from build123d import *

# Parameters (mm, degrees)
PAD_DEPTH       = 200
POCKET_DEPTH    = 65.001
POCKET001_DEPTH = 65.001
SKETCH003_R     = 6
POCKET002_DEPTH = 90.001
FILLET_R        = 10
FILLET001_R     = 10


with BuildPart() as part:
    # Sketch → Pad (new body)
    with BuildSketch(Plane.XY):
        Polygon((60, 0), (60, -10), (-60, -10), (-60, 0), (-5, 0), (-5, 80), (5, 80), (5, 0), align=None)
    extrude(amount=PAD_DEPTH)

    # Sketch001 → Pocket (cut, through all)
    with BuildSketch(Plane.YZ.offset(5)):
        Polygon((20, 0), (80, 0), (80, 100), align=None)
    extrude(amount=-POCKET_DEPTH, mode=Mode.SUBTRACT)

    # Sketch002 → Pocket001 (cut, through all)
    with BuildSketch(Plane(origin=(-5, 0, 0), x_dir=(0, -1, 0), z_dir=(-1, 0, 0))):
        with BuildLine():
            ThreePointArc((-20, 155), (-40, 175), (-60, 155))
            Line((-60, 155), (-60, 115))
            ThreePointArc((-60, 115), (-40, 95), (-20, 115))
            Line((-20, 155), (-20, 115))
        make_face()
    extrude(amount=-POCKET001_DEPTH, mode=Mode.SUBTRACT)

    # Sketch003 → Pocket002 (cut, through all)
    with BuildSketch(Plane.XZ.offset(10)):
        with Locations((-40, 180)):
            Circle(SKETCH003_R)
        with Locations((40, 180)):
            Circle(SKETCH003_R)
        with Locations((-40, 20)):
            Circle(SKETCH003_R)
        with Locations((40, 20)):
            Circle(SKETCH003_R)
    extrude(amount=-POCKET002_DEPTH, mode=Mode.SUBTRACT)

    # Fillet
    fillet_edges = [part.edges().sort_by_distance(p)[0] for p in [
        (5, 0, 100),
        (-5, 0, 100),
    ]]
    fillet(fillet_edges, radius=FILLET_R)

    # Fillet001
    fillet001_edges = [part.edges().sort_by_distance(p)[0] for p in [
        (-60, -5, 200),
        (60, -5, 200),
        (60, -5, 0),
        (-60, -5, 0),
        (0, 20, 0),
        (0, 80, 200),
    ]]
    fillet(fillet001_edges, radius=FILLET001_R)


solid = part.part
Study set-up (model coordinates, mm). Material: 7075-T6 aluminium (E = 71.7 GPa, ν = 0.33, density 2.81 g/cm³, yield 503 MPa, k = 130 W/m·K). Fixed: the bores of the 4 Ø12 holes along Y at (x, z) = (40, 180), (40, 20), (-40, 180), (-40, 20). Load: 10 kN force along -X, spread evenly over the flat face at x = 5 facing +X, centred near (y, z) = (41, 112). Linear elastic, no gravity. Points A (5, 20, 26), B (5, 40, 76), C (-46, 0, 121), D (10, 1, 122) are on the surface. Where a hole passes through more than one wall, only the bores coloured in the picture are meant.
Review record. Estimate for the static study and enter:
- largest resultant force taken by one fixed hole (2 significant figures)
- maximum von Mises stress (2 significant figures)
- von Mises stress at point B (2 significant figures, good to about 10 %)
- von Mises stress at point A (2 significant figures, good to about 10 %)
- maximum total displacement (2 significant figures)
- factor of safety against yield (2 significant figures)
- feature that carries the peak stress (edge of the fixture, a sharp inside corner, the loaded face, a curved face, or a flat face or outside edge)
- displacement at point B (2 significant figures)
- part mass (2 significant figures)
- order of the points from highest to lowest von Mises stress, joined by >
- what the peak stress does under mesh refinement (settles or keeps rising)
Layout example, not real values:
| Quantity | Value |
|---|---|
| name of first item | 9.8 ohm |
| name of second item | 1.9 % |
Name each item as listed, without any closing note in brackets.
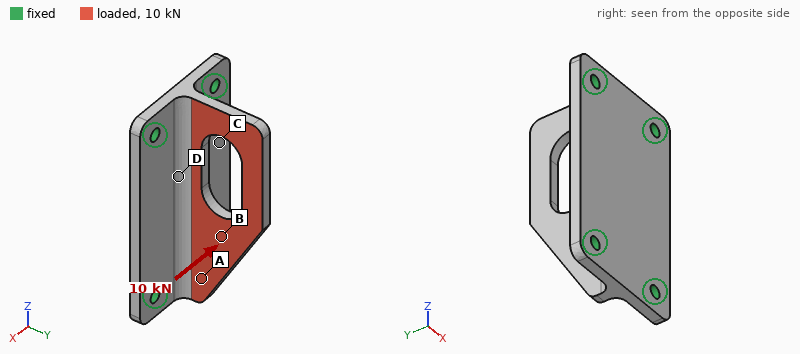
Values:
| Quantity | Value |
|---|---|
| largest resultant force taken by one fixed hole | 5.1 kN |
| maximum von Mises stress | 210 MPa |
| von Mises stress at point B | 87 MPa |
| von Mises stress at point A | 62 MPa |
| maximum total displacement | 1.3 mm |
| factor of safety against yield | 2.4 |
| feature that carries the peak stress | a curved face |
| displacement at point B | 0.34 mm |
| part mass | 970 g |
| order of the points from highest to lowest von Mises stress, joined by > | B > A > D > C |
| what the peak stress does under mesh refinement | settles |
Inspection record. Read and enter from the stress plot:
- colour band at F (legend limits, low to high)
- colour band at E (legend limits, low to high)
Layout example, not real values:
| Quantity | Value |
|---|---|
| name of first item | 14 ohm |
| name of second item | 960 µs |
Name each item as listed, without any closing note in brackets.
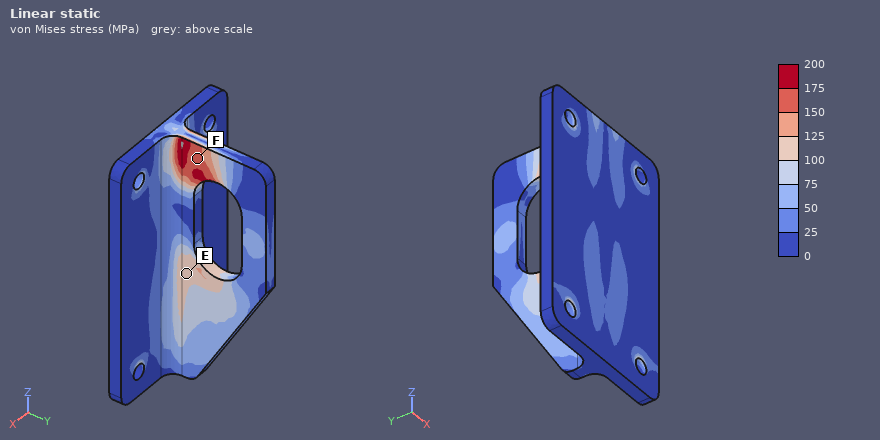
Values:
| Quantity | Value |
|---|---|
| colour band at F | 150 to 175 MPa |
| colour band at E | 100 to 125 MPa |
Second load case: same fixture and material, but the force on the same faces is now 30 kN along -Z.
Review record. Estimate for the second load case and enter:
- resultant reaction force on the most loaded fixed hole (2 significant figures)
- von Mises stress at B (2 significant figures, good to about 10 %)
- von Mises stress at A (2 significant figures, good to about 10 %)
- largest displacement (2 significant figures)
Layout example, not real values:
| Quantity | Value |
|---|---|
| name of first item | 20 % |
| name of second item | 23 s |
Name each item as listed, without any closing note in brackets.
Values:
| Quantity | Value |
|---|---|
| resultant reaction force on the most loaded fixed hole | 9.5 kN |
| von Mises stress at B | 45 MPa |
| von Mises stress at A | 23 MPa |
| largest displacement | 0.32 mm |
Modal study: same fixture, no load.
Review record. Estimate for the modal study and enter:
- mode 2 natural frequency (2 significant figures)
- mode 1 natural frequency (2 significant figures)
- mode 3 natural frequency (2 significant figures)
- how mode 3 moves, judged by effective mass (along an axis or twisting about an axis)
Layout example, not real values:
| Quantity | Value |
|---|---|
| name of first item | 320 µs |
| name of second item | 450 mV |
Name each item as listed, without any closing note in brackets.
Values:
| Quantity | Value |
|---|---|
| mode 2 natural frequency | 2100 Hz |
| mode 1 natural frequency | 1100 Hz |
| mode 3 natural frequency | 2700 Hz |
| how mode 3 moves, judged by effective mass | along Y |
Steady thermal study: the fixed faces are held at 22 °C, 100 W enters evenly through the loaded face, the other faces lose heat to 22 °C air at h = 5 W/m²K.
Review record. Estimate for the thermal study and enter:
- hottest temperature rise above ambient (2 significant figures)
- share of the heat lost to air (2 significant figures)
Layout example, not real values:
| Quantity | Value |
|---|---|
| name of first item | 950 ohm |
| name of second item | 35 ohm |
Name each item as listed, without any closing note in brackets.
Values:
| Quantity | Value |
|---|---|
| hottest temperature rise above ambient | 53 K |
| share of the heat lost to air | 4.2 % |
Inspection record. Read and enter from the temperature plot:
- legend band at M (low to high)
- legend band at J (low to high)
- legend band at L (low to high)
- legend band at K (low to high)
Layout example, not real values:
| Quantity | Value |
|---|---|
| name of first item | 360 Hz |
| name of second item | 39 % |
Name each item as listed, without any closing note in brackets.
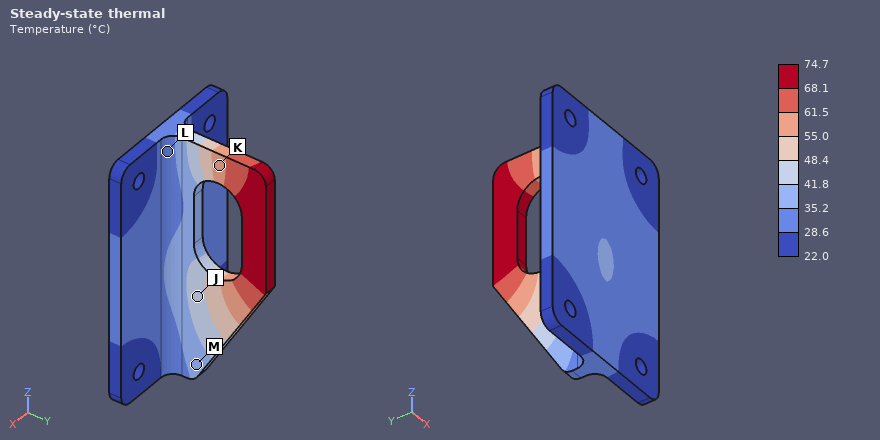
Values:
| Quantity | Value |
|---|---|
| legend band at M | 35.2 to 41.8 °C |
| legend band at J | 41.8 to 48.4 °C |
| legend band at L | 28.6 to 35.2 °C |
| legend band at K | 55.0 to 61.5 °C |
